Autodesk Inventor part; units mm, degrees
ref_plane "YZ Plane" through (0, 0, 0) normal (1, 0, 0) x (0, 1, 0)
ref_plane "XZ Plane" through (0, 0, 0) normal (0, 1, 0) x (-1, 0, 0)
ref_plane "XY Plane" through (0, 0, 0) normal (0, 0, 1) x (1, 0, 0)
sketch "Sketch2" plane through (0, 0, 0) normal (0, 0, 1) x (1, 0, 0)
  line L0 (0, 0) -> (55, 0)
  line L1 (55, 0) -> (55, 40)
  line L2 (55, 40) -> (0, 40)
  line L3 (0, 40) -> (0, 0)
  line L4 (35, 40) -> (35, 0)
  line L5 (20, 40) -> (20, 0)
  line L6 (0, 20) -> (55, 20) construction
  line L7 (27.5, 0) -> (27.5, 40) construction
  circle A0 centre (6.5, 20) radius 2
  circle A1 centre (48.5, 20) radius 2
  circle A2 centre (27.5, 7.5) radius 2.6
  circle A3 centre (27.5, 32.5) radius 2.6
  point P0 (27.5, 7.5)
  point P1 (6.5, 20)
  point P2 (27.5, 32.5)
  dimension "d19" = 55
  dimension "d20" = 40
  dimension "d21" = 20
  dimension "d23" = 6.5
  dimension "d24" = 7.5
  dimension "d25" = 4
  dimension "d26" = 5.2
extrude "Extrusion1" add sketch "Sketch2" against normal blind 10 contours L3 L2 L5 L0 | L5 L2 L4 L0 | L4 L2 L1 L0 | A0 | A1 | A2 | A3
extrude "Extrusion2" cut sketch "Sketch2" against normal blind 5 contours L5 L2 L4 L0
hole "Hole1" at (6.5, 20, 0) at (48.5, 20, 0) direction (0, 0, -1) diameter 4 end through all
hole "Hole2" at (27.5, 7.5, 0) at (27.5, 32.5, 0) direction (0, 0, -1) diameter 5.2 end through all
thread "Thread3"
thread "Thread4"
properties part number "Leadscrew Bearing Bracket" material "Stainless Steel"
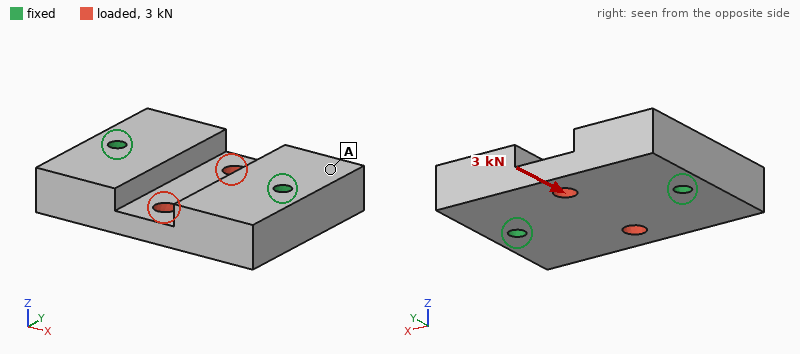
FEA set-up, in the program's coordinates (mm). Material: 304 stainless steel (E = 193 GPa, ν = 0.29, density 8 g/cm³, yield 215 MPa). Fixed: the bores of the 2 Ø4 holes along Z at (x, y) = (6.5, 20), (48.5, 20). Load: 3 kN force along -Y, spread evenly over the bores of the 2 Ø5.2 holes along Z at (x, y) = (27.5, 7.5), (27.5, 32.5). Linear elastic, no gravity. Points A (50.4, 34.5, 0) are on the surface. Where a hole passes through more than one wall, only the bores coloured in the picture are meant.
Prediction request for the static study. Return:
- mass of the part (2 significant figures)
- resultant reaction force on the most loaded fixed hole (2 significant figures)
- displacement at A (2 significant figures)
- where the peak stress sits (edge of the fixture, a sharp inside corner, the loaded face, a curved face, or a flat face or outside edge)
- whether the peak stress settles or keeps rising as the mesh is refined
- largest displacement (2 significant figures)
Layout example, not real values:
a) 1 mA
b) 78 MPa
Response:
a) 150 g
b) 1.5 kN
c) 1.4 µm
d) edge of the fixture
e) keeps rising
f) 4.6 µm
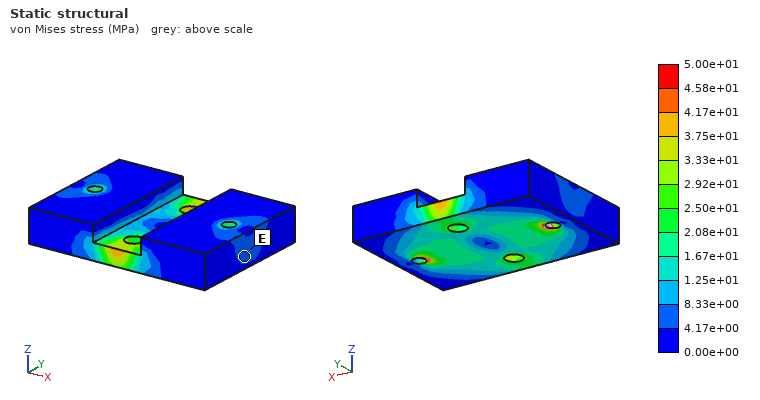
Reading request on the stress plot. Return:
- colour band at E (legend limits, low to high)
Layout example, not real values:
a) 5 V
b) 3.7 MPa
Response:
a) 4.17e+00 to 8.33e+00 MPa
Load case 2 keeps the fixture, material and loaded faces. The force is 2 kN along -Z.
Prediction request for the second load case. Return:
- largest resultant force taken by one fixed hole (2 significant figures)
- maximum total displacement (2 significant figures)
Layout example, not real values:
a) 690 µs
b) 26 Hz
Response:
a) 1.3 kN
b) 8.2 µm
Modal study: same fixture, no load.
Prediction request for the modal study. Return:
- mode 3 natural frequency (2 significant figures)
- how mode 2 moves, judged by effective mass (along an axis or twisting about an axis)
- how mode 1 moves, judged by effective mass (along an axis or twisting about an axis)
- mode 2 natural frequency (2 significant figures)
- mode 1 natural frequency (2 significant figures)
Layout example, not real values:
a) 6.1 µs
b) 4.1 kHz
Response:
a) 16 kHz
b) along Z
c) twisting about X
d) 14 kHz
e) 11 kHz
